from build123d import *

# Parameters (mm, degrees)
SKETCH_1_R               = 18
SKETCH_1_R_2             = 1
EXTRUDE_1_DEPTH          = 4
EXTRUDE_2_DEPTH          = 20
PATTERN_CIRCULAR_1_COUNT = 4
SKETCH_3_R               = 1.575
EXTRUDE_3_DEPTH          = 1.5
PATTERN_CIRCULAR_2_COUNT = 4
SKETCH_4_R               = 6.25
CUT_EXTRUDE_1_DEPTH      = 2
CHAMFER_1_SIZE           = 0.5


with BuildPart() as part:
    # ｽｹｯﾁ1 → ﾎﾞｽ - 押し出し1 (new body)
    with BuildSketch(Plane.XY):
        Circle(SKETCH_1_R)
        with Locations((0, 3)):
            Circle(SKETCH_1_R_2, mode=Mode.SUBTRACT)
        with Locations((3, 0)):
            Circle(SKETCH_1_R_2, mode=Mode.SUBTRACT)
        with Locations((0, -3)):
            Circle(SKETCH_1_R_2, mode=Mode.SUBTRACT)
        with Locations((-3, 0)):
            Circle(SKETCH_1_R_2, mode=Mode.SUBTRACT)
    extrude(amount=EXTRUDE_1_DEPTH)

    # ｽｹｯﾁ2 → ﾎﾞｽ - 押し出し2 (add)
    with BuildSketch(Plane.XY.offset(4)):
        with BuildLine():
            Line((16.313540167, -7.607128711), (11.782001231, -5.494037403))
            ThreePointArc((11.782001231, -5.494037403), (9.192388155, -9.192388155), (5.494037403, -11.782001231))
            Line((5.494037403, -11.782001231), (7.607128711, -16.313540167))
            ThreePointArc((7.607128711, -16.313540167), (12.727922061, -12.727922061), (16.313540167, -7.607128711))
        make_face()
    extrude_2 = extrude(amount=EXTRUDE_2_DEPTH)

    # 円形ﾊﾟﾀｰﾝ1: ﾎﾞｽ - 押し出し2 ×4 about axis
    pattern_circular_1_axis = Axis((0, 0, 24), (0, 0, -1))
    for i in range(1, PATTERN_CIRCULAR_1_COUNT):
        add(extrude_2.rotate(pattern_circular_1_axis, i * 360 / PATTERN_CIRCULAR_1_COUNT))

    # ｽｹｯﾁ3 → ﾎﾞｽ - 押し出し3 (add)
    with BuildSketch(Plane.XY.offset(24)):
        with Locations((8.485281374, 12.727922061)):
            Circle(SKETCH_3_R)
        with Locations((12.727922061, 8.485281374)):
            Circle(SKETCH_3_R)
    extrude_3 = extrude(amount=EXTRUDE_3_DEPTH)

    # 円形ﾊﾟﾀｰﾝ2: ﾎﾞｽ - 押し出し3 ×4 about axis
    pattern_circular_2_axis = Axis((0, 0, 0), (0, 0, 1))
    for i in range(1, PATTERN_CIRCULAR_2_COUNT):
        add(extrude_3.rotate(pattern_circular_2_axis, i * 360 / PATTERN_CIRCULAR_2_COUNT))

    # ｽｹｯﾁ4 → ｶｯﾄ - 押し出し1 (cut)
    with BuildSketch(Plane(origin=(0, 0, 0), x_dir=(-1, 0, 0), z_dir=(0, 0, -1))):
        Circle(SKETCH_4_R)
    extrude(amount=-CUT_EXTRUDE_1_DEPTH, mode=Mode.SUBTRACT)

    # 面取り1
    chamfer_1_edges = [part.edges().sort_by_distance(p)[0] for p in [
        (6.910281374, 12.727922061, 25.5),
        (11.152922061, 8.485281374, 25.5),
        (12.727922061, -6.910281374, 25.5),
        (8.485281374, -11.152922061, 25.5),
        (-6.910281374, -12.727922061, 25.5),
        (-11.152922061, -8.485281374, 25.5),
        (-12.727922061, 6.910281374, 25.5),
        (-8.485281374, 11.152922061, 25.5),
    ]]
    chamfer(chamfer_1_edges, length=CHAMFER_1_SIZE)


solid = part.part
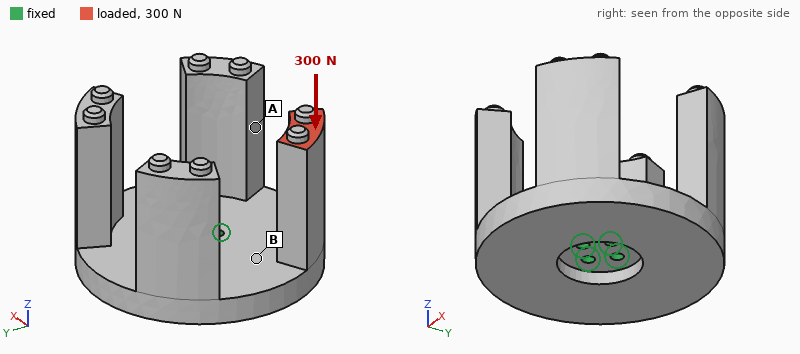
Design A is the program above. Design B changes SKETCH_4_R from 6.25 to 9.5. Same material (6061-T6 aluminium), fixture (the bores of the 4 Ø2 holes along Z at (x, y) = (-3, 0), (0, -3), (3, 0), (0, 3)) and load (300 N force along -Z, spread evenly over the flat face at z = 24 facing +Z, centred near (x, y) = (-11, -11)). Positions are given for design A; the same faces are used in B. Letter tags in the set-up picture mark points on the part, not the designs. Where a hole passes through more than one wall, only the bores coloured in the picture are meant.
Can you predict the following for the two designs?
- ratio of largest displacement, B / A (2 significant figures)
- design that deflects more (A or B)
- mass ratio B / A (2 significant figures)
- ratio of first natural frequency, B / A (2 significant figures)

1.3
B
0.96
0.86
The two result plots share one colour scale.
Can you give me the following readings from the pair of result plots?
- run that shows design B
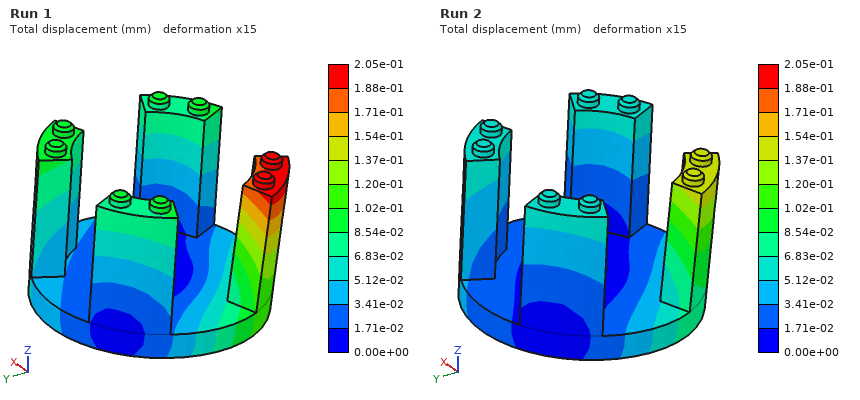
Run 1
